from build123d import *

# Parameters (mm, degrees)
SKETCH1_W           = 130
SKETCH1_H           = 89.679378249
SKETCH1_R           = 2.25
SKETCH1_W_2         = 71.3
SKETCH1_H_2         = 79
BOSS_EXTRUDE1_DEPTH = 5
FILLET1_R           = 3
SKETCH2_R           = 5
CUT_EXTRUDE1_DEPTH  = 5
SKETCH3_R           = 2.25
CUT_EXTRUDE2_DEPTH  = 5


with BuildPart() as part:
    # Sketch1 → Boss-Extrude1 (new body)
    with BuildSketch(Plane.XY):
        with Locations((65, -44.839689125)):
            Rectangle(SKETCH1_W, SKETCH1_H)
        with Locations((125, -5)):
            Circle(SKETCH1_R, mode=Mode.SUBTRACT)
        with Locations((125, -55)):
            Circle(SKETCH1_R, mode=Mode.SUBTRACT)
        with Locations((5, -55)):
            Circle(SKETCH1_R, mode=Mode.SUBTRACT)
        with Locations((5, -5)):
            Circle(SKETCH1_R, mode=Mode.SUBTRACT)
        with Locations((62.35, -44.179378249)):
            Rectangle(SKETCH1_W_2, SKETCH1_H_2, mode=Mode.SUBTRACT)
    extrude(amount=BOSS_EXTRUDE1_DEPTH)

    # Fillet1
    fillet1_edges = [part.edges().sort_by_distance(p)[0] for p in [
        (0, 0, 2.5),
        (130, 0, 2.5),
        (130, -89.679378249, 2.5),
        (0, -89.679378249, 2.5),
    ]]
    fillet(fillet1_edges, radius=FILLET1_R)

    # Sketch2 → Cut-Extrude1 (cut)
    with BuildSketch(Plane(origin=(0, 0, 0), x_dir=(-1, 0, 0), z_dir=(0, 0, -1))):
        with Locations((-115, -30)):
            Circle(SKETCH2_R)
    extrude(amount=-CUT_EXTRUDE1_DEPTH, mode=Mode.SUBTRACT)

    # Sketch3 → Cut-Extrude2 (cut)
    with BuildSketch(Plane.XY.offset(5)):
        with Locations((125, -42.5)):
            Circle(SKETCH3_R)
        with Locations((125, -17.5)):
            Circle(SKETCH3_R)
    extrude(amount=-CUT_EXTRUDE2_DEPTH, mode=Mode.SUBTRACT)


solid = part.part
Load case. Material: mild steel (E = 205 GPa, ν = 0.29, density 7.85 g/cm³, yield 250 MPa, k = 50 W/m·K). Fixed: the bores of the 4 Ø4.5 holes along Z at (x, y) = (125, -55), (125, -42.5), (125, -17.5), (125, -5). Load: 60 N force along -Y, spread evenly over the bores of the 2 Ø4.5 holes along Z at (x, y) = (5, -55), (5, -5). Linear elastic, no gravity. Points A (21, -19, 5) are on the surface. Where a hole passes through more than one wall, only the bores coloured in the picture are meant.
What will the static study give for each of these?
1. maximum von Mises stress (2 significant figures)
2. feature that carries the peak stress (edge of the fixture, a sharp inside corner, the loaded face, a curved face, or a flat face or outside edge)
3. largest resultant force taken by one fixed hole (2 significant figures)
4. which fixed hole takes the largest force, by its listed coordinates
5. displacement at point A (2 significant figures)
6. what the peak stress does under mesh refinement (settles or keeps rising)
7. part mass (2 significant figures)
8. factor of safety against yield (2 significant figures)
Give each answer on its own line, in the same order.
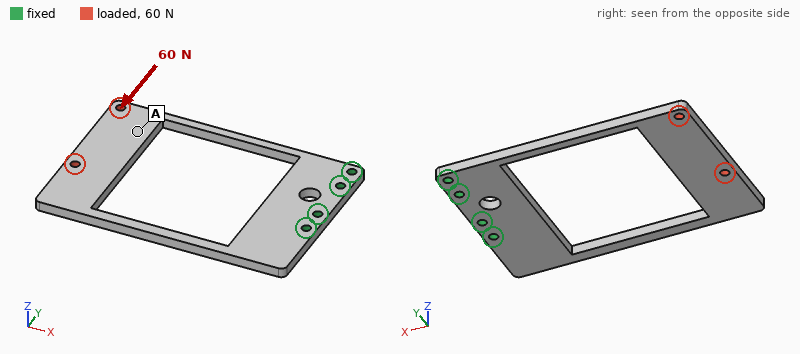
47 MPa
a flat face or outside edge
170 N
(125, -55)
92 µm
settles
230 g
5.4
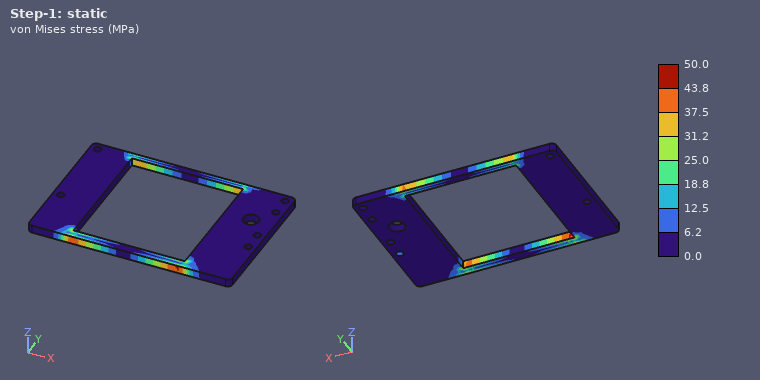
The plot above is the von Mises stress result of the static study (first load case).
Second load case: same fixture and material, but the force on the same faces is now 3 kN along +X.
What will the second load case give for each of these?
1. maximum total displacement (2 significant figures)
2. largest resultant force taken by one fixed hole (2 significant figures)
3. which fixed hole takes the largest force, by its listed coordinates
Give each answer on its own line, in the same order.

48 µm
1.8 kN
(125, -55)
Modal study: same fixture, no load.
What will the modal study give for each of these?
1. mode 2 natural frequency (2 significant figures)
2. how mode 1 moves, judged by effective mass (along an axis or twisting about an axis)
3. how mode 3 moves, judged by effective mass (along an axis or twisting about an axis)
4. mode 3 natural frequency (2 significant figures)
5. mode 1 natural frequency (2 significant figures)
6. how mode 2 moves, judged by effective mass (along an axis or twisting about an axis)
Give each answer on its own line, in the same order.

400 Hz
along Z
twisting about X
470 Hz
140 Hz
along Y
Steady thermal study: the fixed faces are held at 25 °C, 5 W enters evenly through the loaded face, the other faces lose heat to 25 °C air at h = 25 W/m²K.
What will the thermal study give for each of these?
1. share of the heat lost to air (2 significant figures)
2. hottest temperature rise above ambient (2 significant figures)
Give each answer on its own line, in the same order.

92 %
36 K
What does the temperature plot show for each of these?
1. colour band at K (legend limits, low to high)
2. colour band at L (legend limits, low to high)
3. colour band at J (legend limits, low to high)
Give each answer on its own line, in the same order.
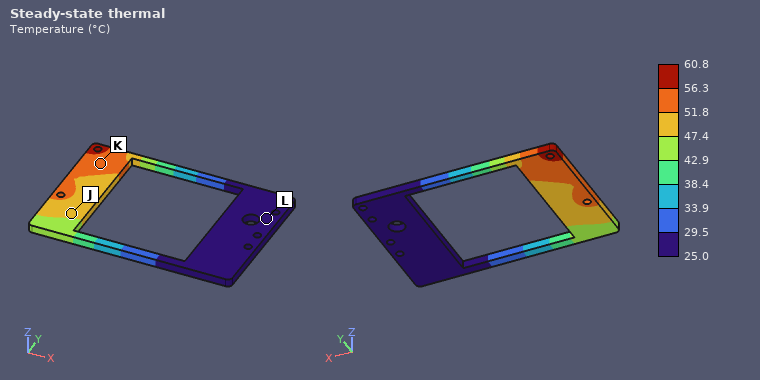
51.8 to 56.3 °C
25.0 to 29.5 °C
47.4 to 51.8 °C
